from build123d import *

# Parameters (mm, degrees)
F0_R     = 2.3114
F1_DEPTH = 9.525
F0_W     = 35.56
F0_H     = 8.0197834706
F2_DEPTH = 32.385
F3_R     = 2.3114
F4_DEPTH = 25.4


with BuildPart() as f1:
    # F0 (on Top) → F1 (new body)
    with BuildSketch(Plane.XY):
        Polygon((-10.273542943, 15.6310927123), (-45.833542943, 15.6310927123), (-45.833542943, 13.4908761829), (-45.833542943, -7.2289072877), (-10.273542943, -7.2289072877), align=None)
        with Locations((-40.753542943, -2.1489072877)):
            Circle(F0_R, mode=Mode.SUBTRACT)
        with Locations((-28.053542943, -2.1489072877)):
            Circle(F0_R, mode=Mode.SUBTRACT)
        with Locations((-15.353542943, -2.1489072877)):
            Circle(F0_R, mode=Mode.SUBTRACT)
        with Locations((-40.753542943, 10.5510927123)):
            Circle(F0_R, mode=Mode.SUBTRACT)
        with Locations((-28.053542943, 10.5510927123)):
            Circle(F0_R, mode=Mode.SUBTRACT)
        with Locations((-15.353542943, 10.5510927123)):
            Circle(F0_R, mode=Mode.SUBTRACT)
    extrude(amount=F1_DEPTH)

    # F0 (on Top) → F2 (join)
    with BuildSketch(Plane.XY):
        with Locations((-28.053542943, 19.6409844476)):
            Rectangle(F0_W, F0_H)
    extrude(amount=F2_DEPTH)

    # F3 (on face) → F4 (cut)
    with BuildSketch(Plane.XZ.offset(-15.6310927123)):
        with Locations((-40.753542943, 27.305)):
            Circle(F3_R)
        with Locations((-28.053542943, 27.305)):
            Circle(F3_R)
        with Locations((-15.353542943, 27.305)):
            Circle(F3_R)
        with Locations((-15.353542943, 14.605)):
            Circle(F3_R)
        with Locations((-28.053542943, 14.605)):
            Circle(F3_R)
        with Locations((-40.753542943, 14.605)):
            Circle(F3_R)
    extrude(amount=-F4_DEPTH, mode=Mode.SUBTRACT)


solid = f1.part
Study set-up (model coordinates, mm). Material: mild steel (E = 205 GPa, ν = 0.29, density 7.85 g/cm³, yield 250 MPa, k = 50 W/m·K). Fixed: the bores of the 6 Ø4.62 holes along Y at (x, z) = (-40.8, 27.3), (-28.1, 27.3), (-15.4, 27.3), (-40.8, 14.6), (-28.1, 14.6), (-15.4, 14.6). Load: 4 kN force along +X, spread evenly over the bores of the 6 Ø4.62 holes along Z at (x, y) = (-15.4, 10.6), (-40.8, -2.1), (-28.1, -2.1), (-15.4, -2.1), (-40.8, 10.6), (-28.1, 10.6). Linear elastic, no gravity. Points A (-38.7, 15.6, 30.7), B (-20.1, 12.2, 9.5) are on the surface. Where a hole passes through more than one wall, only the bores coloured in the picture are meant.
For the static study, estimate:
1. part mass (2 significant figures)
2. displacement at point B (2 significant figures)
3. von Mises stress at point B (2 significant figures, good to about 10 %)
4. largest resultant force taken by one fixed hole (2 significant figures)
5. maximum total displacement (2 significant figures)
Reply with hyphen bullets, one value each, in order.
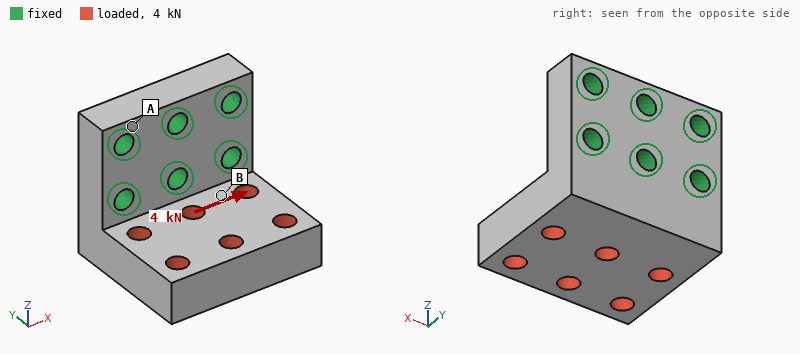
- 120 g
- 4.8 µm
- 53 MPa
- 2.7 kN
- 16 µm
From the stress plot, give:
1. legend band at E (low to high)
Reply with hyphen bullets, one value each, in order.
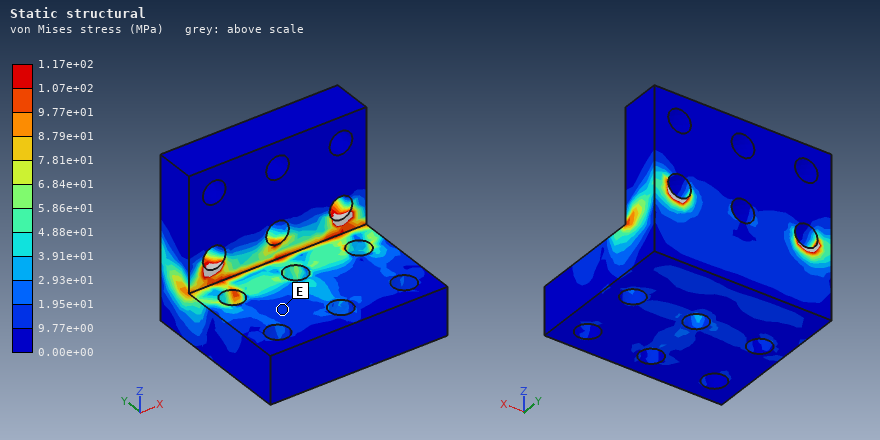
- 9.77e+00 to 1.95e+01 MPa
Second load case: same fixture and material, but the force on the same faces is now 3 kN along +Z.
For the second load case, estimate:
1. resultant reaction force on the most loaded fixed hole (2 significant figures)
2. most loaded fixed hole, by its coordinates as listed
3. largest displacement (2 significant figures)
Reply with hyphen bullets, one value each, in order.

- 1.1 kN
- (-28.1, 14.6)
- 47 µm
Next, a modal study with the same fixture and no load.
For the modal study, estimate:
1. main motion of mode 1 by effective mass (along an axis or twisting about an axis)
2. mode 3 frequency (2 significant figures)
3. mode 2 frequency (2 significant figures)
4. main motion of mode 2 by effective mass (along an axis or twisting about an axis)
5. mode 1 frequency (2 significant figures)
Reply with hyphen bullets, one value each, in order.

- along Z
- 16 kHz
- 12 kHz
- along X
- 6500 Hz
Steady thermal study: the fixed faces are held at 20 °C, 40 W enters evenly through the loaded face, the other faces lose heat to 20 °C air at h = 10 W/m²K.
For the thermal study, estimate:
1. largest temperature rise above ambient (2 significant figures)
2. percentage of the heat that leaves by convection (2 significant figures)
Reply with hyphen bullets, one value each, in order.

- 59 K
- 3.0 %
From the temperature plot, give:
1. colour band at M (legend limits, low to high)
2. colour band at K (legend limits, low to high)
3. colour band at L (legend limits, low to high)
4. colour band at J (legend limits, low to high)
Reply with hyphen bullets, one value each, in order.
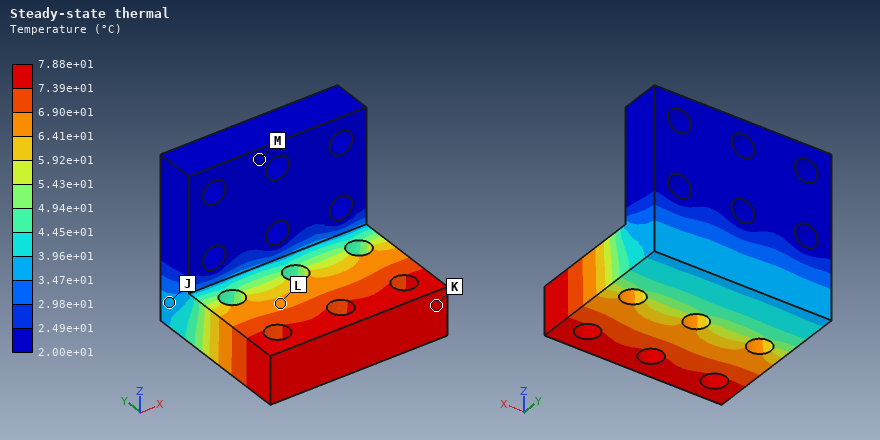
- 2.00e+01 to 2.49e+01 °C
- 7.39e+01 to 7.88e+01 °C
- 6.41e+01 to 6.90e+01 °C
- 3.47e+01 to 3.96e+01 °C
